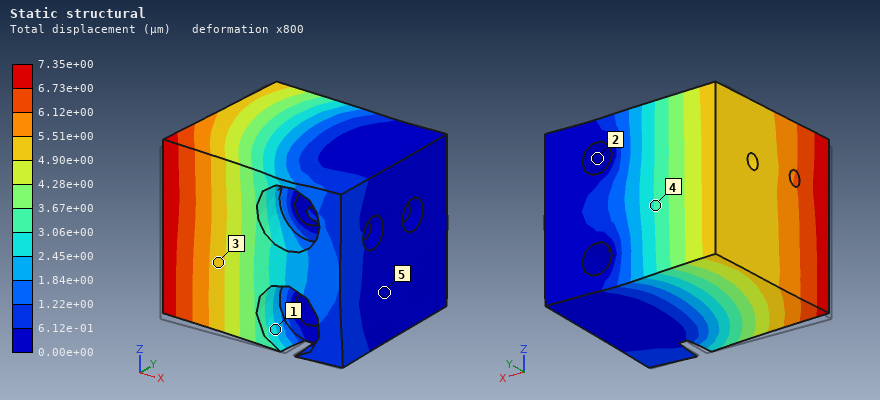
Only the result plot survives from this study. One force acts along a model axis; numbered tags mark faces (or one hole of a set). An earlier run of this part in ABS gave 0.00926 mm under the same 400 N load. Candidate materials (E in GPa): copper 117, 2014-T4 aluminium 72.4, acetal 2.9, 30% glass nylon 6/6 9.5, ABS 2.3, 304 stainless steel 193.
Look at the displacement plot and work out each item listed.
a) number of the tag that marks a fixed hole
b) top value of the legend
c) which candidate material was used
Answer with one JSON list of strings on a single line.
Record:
["2", "7.35e+00 µm", "acetal"]
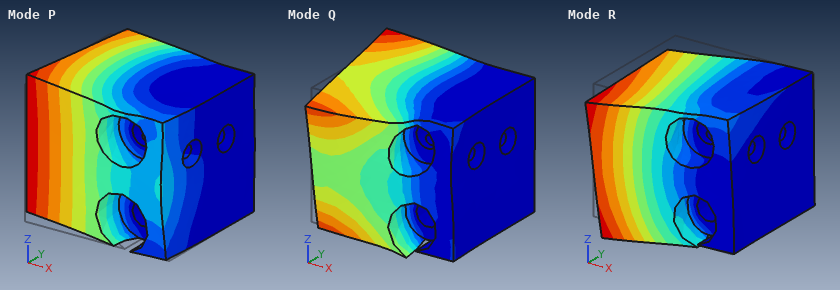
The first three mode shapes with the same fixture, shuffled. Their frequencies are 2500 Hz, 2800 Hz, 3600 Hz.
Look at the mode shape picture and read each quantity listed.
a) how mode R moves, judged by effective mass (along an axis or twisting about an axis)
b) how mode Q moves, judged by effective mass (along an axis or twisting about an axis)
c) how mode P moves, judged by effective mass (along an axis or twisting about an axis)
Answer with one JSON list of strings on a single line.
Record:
["along Z", "twisting about X", "along Y"]
